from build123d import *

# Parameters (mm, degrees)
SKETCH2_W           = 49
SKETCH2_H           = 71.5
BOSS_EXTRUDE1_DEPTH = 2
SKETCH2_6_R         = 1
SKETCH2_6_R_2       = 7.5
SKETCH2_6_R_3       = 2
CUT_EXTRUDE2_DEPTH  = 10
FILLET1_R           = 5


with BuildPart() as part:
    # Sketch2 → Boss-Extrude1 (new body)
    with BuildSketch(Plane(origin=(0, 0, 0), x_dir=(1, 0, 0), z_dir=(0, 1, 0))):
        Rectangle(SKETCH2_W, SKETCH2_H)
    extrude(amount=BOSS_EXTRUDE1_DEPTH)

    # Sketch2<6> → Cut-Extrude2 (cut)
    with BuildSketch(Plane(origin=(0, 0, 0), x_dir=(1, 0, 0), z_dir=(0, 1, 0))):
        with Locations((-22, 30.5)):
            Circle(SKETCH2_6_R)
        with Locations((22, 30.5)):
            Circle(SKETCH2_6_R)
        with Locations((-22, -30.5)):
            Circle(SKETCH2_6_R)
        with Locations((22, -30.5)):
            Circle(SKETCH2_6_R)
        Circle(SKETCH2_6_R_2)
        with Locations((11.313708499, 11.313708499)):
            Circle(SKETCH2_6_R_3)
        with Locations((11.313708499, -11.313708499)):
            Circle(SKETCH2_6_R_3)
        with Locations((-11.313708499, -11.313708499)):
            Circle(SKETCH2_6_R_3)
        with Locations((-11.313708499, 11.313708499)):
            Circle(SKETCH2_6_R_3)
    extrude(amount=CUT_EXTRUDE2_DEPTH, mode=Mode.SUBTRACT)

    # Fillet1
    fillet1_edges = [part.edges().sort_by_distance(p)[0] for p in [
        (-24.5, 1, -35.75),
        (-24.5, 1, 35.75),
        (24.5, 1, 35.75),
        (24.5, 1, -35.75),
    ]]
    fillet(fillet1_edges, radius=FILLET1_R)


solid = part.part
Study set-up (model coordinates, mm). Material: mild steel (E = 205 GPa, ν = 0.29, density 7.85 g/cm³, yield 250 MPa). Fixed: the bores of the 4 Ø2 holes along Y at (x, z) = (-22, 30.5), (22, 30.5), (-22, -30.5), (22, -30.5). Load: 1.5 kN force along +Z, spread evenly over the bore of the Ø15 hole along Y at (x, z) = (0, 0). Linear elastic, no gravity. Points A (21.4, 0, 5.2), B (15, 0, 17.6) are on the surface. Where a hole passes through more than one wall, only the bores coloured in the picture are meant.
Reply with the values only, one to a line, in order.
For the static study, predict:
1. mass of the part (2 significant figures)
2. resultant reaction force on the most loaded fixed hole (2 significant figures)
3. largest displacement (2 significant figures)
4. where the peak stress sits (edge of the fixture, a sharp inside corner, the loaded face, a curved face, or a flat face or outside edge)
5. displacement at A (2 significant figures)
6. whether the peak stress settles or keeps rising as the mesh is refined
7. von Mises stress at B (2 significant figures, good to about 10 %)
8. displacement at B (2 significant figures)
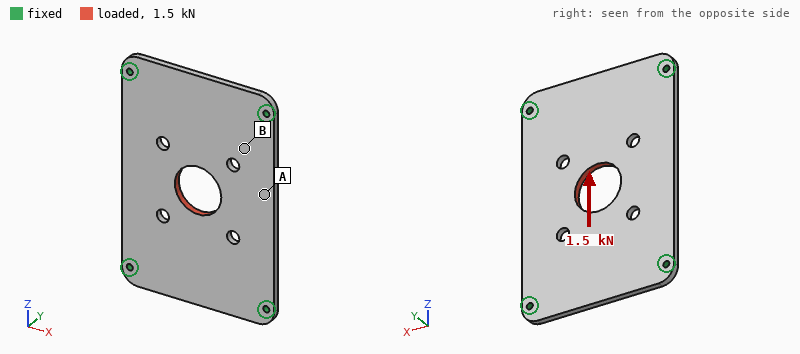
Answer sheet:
51 g
400 N
3.0 µm
edge of the fixture
1.6 µm
keeps rising
11 MPa
1.5 µm
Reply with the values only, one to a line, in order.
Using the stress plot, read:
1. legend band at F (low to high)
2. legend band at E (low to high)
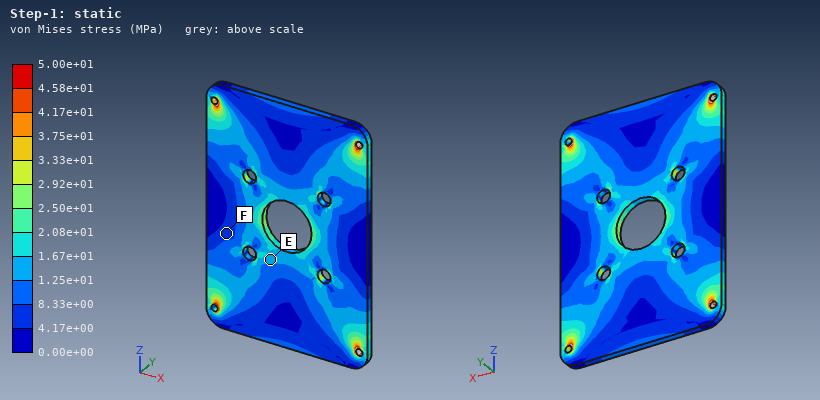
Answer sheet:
4.17e+00 to 8.33e+00 MPa
1.25e+01 to 1.67e+01 MPa
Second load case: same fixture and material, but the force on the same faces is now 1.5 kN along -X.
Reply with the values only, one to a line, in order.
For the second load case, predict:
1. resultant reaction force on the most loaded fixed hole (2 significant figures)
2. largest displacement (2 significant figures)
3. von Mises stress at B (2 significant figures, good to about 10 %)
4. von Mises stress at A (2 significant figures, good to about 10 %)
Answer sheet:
450 N
4.6 µm
14 MPa
11 MPa
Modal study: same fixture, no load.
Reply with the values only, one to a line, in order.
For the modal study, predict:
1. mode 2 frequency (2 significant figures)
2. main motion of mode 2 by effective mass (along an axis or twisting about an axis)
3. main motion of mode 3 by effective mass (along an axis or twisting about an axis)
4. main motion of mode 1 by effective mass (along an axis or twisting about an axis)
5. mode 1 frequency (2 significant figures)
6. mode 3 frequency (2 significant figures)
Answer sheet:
3500 Hz
twisting about Z
twisting about X
along Y
2100 Hz
4700 Hz
